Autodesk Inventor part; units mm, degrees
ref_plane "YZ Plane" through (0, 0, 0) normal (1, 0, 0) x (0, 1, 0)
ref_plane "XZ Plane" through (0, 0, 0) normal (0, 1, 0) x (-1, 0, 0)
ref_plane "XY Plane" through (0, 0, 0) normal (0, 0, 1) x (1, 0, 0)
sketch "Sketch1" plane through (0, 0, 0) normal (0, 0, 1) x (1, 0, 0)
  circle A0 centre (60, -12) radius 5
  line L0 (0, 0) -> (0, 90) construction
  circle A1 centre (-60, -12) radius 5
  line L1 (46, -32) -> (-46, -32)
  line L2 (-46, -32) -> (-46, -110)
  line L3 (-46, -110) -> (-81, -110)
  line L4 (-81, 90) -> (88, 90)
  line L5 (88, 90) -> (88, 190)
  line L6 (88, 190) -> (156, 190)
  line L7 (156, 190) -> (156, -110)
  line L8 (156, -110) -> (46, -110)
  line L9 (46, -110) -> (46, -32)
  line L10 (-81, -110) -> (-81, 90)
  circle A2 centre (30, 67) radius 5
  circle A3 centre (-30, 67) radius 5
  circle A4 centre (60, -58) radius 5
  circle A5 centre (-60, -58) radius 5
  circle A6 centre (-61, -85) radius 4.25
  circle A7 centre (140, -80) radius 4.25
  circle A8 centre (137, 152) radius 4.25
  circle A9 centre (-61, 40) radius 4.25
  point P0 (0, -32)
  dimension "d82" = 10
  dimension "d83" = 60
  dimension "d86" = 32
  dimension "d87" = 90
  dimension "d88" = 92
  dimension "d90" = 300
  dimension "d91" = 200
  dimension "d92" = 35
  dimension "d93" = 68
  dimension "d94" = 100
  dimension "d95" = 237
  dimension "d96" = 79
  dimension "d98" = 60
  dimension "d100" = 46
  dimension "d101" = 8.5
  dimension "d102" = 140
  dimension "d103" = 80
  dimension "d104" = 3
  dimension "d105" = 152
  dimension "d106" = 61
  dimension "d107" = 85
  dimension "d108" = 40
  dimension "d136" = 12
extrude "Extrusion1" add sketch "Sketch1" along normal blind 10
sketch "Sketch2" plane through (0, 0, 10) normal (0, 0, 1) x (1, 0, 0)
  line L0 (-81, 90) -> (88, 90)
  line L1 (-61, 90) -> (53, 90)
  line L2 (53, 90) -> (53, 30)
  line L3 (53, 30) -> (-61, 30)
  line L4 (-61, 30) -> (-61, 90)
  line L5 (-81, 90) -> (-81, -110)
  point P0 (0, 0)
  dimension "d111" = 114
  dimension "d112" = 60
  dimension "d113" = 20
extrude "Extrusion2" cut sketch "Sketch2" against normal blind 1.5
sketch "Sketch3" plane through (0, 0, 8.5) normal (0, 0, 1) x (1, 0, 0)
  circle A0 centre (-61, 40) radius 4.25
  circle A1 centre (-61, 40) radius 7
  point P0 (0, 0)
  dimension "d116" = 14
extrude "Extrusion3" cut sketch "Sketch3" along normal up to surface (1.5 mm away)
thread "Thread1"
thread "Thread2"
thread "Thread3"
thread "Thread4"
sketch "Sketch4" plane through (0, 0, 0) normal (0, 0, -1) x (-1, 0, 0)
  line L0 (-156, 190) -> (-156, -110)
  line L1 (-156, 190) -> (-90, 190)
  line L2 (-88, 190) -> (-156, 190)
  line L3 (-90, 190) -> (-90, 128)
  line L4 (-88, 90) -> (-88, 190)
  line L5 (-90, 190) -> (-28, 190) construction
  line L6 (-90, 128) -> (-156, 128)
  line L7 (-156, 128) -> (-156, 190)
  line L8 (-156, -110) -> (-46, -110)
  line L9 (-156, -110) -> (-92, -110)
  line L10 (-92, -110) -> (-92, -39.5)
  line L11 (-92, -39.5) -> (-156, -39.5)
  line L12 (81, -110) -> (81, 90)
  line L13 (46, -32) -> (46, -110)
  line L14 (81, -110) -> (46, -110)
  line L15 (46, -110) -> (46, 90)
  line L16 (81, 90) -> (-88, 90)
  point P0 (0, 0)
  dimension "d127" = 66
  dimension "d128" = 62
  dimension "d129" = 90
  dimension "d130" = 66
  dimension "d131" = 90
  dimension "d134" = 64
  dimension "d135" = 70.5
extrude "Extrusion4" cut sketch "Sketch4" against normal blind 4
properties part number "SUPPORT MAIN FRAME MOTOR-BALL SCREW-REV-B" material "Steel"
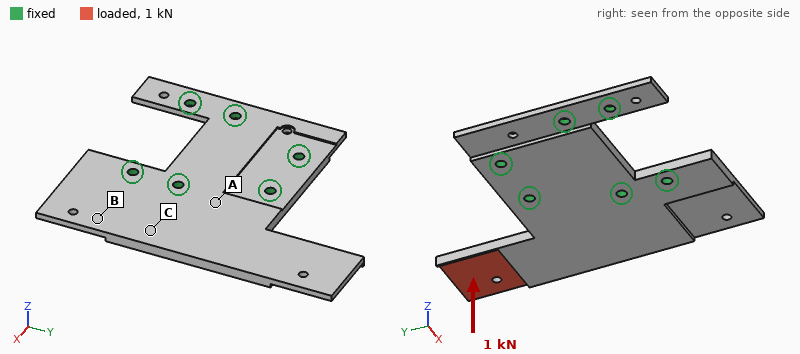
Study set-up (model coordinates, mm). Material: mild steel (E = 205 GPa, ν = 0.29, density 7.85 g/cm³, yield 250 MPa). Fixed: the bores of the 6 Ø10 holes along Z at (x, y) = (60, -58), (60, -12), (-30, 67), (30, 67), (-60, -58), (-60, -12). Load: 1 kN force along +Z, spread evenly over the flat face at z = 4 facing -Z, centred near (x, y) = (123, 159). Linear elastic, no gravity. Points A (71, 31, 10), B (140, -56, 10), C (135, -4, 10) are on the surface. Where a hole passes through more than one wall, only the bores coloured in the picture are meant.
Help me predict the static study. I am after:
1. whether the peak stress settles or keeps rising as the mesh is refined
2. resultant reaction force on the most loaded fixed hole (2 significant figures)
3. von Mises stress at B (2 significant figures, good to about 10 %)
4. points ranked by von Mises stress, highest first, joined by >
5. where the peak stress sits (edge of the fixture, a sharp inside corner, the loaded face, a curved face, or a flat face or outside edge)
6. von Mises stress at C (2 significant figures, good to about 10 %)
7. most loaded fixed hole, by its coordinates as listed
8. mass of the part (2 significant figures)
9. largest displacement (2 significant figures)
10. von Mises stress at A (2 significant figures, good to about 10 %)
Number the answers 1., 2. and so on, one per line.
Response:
1. keeps rising
2. 1.6 kN
3. 14 MPa
4. A > C > B
5. edge of the fixture
6. 27 MPa
7. (30, 67)
8. 3.1 kg
9. 1.1 mm
10. 45 MPa
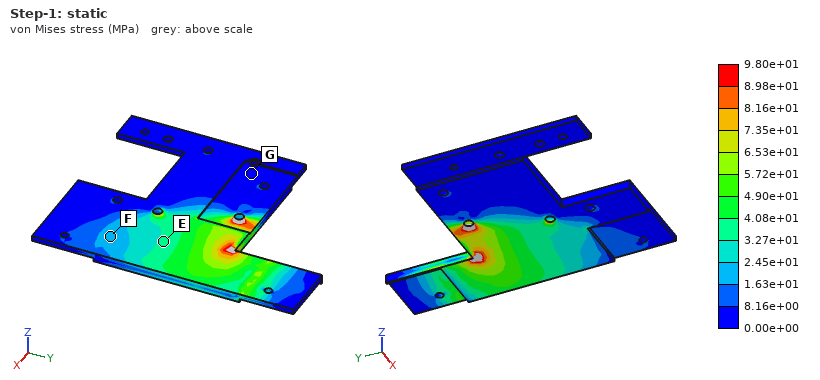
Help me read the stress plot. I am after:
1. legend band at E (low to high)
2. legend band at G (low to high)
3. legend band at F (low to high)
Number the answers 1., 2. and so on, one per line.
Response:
1. 3.27e+01 to 4.08e+01 MPa
2. 0.00e+00 to 8.16e+00 MPa
3. 1.63e+01 to 2.45e+01 MPa
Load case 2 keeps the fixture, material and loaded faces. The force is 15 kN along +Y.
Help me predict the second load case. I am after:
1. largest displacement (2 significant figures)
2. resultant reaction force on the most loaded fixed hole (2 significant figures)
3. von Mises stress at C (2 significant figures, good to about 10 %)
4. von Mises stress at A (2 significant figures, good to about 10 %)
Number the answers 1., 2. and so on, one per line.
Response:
1. 0.38 mm
2. 8.6 kN
3. 11 MPa
4. 15 MPa
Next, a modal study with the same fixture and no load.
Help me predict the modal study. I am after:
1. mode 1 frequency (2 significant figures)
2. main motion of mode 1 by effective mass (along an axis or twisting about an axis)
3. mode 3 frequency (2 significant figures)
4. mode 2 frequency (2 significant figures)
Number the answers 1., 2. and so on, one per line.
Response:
1. 340 Hz
2. along Z
3. 1100 Hz
4. 780 Hz
